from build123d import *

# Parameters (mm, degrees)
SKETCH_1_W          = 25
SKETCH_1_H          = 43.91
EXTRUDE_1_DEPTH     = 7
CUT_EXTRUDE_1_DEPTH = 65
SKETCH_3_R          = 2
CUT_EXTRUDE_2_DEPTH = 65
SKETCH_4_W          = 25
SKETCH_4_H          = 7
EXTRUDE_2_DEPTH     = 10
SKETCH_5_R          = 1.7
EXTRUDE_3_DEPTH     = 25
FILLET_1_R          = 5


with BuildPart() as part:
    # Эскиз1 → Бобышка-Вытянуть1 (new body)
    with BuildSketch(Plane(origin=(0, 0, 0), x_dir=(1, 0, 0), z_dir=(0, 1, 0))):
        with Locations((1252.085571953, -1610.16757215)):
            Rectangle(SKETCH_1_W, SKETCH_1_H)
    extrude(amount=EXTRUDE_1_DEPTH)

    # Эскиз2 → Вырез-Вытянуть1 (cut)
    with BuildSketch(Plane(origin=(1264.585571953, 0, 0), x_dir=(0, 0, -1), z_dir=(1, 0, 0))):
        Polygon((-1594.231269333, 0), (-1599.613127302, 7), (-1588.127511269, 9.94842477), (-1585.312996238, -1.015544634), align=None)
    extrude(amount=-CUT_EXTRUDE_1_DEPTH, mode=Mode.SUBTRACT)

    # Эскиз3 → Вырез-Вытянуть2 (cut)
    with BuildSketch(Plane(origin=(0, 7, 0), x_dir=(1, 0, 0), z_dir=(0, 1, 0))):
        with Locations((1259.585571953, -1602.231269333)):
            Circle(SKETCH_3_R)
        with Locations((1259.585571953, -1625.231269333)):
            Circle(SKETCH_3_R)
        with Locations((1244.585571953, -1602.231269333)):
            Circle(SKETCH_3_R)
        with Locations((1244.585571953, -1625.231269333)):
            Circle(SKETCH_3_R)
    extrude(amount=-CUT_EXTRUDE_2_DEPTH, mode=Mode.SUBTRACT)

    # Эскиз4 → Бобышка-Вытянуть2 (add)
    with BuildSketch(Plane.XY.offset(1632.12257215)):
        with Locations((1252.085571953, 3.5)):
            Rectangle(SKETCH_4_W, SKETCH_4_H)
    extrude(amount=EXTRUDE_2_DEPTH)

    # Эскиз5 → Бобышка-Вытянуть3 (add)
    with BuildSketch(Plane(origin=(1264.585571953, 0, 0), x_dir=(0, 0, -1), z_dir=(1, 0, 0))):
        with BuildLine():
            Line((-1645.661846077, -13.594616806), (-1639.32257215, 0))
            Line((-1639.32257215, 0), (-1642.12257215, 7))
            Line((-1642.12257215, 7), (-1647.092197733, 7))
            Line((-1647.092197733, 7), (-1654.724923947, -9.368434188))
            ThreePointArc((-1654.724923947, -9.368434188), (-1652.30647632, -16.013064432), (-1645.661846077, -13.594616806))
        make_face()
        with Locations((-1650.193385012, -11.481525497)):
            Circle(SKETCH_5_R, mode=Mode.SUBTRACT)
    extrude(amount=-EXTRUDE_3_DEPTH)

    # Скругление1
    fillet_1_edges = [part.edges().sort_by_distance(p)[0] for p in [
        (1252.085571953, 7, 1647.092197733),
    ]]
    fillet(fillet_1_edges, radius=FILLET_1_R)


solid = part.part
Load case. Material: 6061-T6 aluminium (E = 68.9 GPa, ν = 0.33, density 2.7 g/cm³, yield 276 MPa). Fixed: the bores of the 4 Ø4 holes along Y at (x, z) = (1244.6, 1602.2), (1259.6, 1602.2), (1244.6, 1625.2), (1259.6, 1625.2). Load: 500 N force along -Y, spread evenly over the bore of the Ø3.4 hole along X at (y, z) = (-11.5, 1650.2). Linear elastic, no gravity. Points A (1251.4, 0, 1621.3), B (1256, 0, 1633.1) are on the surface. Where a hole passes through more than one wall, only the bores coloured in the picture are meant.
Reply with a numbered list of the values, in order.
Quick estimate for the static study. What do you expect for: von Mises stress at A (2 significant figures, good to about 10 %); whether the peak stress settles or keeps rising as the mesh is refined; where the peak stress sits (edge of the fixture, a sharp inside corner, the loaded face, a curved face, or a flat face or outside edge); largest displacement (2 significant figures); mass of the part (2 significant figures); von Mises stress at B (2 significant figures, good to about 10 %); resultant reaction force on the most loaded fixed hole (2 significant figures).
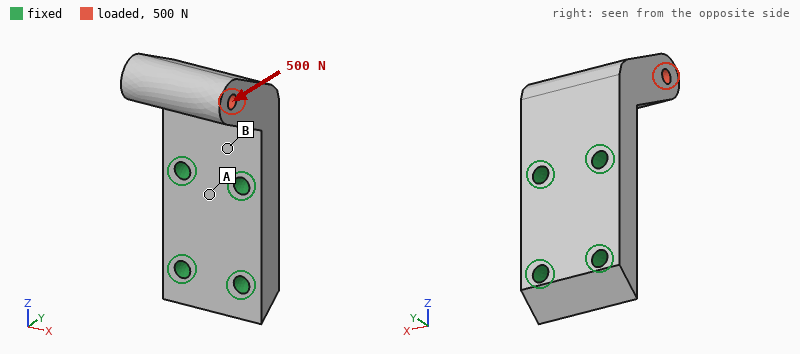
1. 12 MPa
2. keeps rising
3. edge of the fixture
4. 81 µm
5. 34 g
6. 38 MPa
7. 290 N
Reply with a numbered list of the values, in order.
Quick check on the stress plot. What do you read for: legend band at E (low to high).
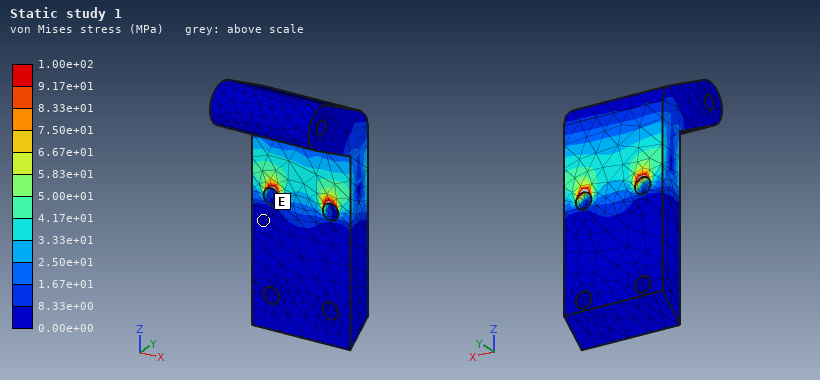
1. 0.00e+00 to 8.33e+00 MPa
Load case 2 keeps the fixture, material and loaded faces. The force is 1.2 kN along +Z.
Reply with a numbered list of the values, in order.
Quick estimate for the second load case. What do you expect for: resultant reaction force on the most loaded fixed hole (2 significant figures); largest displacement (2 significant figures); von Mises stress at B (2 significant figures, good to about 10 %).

1. 580 N
2. 0.17 mm
3. 88 MPa
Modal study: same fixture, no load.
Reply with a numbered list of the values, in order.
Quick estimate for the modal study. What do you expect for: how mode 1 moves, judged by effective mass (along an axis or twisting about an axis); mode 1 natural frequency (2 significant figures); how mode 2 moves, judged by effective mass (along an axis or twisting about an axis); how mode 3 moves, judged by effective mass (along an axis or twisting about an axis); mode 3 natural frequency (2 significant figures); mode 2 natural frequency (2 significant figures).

1. along Y
2. 4000 Hz
3. along X
4. along X
5. 15 kHz
6. 7700 Hz
